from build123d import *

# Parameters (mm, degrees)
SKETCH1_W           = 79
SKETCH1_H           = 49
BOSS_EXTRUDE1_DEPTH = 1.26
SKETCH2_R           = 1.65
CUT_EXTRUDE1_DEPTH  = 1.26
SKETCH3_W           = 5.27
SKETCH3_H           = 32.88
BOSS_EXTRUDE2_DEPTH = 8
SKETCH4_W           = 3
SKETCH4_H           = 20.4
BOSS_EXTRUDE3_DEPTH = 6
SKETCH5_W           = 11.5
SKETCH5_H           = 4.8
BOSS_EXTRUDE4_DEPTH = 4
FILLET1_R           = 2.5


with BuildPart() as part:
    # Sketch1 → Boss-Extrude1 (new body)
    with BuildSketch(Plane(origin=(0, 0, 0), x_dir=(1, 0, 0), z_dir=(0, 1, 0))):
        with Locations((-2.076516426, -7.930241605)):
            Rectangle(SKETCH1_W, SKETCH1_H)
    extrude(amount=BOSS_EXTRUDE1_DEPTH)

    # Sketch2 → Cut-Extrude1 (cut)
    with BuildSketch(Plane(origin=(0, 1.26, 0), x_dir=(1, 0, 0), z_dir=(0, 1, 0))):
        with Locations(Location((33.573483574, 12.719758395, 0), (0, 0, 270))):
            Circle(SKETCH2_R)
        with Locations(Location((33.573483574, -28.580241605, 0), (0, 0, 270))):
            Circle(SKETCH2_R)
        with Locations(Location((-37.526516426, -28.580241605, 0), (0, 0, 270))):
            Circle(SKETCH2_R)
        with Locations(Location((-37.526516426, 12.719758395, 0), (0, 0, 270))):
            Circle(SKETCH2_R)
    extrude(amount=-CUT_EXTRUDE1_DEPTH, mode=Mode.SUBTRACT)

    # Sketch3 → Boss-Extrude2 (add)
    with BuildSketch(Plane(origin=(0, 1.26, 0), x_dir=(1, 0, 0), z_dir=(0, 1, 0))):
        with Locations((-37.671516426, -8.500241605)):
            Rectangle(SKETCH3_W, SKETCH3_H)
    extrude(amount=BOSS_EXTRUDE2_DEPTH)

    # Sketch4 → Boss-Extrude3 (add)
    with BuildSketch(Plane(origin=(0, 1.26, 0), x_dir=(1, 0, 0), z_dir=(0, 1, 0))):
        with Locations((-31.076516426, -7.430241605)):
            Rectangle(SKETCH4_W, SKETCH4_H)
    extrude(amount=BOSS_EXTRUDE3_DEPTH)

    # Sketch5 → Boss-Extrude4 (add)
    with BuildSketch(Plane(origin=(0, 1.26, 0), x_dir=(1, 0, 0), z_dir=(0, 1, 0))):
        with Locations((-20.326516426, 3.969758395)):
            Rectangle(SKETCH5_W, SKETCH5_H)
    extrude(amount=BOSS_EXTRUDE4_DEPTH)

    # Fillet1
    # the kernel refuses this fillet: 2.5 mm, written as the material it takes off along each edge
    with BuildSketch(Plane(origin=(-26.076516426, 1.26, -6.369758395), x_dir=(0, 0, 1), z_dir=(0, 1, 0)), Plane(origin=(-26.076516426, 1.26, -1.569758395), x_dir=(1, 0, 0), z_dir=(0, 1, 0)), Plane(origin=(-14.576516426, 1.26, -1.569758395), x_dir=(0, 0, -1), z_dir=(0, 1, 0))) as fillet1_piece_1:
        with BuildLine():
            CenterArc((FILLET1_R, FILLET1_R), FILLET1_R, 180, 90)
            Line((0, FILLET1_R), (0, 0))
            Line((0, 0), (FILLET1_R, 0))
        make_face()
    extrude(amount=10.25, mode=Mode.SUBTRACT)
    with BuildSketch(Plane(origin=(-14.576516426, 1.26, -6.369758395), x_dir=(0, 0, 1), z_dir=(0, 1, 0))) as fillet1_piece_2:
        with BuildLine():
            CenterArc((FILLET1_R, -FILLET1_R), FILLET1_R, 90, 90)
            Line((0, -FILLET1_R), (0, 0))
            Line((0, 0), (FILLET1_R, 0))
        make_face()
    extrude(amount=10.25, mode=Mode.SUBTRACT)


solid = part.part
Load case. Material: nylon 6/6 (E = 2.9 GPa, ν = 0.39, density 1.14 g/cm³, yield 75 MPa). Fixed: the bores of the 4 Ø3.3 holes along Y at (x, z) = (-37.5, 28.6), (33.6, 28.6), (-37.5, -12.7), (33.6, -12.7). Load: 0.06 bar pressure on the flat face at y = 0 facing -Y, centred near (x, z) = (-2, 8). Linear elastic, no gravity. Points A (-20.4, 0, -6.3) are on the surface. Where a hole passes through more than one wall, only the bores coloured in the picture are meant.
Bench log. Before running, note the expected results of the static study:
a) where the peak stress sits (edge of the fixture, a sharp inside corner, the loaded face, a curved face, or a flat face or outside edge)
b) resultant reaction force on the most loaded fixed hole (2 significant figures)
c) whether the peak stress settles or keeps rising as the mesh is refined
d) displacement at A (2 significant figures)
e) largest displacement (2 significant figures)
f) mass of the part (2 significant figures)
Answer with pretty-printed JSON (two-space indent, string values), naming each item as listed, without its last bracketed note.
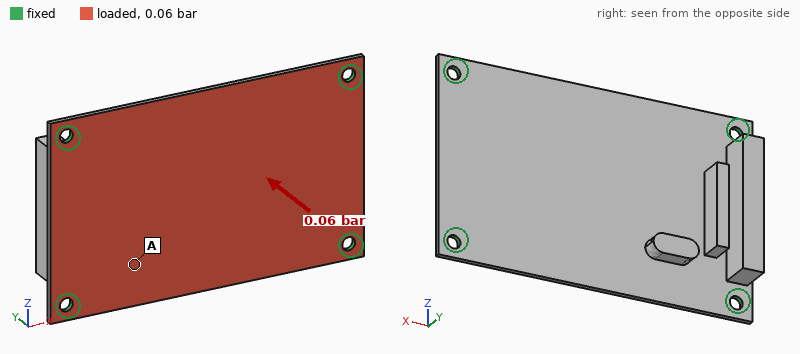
{
  "where the peak stress sits": "edge of the fixture",
  "resultant reaction force on the most loaded fixed hole": "6.7 N",
  "whether the peak stress settles or keeps rising as the mesh is refined": "keeps rising",
  "displacement at A": "0.45 mm",
  "largest displacement": "0.91 mm",
  "mass of the part": "7.7 g"
}
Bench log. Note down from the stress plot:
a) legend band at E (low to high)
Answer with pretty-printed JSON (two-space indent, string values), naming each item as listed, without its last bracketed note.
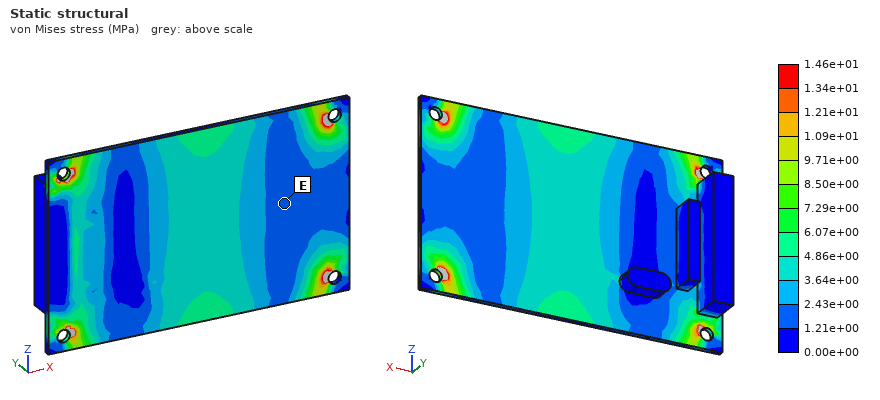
{
  "legend band at E": "1.21e+00 to 2.43e+00 MPa"
}
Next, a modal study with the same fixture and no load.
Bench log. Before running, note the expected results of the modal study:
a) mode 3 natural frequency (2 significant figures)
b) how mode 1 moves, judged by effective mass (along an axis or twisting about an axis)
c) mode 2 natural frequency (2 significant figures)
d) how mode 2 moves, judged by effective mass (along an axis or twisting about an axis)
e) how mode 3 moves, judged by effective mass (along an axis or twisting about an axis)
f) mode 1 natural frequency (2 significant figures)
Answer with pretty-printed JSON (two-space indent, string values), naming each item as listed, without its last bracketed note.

{
  "mode 3 natural frequency": "1000 Hz",
  "how mode 1 moves, judged by effective mass": "along Y",
  "mode 2 natural frequency": "620 Hz",
  "how mode 2 moves, judged by effective mass": "twisting about X",
  "how mode 3 moves, judged by effective mass": "twisting about Z",
  "mode 1 natural frequency": "390 Hz"
}
